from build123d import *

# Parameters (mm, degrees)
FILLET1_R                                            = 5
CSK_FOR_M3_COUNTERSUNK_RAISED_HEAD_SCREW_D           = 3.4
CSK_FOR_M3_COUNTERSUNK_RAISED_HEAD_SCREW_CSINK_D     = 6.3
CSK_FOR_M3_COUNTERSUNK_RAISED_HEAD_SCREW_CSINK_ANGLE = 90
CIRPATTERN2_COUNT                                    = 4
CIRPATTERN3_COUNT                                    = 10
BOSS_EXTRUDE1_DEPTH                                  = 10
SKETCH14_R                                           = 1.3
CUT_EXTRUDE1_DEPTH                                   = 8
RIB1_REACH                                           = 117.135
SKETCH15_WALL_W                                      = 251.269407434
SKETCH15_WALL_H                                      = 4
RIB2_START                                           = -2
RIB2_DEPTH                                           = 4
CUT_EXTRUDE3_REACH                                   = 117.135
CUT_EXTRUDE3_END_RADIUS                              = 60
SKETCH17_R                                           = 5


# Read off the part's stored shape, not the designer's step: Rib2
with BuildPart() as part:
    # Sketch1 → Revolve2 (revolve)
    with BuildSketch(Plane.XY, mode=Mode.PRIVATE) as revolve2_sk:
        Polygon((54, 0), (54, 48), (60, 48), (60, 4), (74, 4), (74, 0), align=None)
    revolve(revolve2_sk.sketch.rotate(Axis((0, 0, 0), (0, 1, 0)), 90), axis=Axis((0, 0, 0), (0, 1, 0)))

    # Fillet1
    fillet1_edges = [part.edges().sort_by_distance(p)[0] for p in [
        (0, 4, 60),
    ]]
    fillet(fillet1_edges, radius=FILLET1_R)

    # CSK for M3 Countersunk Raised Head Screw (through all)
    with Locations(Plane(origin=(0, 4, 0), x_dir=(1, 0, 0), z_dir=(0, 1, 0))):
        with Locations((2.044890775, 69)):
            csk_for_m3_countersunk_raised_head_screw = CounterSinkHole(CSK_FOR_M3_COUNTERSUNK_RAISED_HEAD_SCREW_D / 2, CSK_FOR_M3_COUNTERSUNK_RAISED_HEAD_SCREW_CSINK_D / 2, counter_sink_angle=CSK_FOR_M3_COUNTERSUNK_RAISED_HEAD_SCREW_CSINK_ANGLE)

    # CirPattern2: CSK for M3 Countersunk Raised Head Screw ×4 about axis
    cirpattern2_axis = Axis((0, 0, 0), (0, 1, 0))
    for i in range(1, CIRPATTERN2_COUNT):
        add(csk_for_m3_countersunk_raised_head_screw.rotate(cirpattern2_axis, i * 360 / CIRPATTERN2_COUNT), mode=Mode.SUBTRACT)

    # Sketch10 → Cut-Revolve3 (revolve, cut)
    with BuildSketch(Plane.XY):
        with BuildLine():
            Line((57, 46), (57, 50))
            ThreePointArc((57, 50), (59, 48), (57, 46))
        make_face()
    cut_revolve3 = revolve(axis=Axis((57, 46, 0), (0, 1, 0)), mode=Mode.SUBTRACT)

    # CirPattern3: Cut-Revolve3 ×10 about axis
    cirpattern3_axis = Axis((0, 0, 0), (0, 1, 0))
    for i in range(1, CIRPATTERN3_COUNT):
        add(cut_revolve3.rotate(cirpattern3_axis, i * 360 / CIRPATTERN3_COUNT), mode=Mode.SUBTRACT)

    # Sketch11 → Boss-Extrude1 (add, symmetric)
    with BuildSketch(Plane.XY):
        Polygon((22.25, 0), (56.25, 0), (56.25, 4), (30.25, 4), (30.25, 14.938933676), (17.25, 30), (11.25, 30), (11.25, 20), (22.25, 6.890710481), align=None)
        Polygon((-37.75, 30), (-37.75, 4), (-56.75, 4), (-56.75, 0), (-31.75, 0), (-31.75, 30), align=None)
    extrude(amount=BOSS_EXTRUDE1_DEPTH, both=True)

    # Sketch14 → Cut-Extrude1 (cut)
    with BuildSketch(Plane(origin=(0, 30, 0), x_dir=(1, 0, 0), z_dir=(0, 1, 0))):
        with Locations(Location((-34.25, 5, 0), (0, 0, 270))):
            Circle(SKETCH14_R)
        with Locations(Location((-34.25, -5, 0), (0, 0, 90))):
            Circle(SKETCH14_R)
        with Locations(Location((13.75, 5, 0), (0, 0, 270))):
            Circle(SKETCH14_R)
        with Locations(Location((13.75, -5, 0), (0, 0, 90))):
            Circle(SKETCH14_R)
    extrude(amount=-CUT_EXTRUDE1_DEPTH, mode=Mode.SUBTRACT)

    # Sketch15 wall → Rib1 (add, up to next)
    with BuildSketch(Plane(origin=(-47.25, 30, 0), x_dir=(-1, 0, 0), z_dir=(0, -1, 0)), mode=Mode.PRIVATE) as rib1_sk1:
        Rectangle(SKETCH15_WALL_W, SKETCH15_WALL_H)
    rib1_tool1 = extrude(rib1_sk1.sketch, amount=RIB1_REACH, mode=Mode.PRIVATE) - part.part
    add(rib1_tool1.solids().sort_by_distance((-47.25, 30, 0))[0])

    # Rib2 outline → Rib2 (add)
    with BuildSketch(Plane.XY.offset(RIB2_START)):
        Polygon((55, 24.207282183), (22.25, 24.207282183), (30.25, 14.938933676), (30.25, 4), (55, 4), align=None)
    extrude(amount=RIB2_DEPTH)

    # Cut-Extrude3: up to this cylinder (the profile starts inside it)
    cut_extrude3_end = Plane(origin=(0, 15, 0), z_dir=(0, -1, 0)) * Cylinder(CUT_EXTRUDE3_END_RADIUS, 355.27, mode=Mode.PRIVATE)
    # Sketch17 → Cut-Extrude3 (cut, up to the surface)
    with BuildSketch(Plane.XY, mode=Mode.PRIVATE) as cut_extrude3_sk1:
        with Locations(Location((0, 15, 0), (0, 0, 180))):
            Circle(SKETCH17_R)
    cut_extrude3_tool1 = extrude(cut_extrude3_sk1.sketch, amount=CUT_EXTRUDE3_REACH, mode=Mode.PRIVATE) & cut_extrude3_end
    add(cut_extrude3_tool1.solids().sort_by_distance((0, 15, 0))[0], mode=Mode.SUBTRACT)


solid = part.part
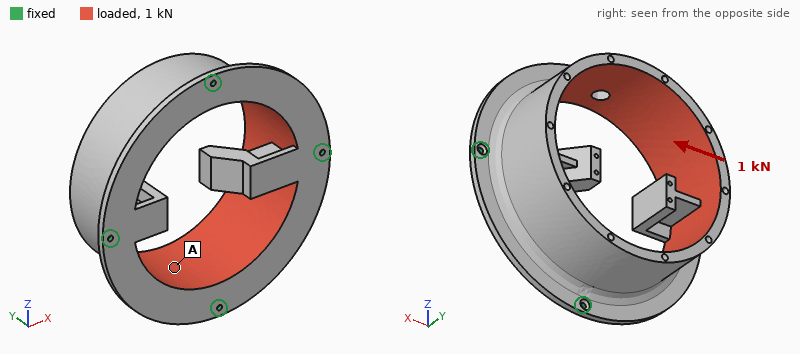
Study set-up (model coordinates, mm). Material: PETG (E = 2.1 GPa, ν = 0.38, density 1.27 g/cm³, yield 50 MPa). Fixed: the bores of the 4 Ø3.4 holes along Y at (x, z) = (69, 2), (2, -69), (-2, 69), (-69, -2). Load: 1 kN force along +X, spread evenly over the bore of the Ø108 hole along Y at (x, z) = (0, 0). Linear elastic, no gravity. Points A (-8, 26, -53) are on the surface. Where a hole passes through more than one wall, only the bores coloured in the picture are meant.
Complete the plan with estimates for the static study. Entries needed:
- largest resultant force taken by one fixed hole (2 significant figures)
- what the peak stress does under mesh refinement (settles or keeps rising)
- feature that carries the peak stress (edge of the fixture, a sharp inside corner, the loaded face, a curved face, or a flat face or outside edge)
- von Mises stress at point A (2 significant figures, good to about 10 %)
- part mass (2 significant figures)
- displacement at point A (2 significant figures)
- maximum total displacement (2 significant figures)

310 N
keeps rising
edge of the fixture
1.1 MPa
180 g
0.14 mm
0.25 mm
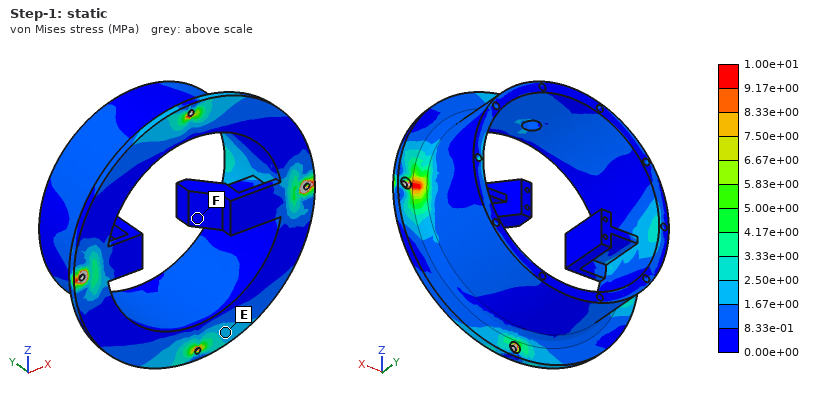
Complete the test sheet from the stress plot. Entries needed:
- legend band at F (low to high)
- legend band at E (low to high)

0.00e+00 to 8.33e-01 MPa
1.67e+00 to 2.50e+00 MPa
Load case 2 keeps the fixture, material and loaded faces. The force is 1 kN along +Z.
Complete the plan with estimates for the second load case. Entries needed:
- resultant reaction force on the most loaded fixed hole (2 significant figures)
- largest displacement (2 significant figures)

310 N
0.25 mm
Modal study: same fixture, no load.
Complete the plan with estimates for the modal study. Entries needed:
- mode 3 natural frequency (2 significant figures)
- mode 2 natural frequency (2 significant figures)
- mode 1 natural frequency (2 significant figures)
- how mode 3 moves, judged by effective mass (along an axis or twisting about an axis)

650 Hz
570 Hz
430 Hz
along Y
